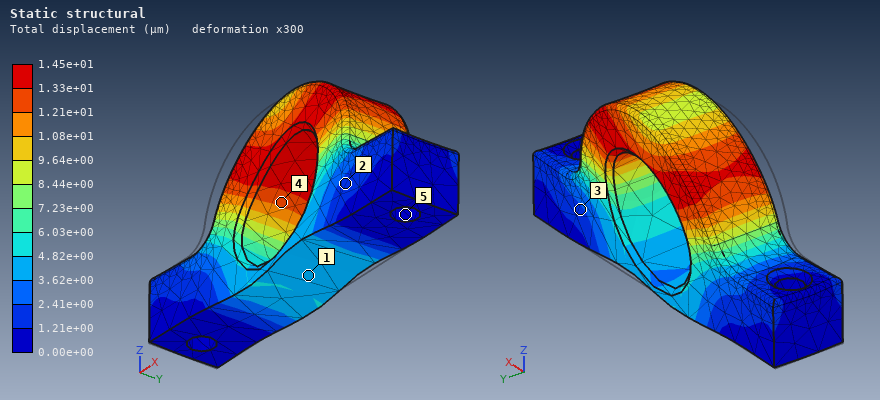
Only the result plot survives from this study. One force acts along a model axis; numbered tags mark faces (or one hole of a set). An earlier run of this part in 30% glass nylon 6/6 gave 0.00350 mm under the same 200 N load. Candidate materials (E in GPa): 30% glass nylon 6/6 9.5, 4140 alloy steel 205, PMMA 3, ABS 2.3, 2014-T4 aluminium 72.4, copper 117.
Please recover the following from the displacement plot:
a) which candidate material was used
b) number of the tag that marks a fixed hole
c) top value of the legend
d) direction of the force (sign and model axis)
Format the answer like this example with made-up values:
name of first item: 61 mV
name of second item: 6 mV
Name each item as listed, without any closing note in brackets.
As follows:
which candidate material was used: ABS
number of the tag that marks a fixed hole: 5
top value of the legend: 1.45e+01 µm
direction of the force: +X
